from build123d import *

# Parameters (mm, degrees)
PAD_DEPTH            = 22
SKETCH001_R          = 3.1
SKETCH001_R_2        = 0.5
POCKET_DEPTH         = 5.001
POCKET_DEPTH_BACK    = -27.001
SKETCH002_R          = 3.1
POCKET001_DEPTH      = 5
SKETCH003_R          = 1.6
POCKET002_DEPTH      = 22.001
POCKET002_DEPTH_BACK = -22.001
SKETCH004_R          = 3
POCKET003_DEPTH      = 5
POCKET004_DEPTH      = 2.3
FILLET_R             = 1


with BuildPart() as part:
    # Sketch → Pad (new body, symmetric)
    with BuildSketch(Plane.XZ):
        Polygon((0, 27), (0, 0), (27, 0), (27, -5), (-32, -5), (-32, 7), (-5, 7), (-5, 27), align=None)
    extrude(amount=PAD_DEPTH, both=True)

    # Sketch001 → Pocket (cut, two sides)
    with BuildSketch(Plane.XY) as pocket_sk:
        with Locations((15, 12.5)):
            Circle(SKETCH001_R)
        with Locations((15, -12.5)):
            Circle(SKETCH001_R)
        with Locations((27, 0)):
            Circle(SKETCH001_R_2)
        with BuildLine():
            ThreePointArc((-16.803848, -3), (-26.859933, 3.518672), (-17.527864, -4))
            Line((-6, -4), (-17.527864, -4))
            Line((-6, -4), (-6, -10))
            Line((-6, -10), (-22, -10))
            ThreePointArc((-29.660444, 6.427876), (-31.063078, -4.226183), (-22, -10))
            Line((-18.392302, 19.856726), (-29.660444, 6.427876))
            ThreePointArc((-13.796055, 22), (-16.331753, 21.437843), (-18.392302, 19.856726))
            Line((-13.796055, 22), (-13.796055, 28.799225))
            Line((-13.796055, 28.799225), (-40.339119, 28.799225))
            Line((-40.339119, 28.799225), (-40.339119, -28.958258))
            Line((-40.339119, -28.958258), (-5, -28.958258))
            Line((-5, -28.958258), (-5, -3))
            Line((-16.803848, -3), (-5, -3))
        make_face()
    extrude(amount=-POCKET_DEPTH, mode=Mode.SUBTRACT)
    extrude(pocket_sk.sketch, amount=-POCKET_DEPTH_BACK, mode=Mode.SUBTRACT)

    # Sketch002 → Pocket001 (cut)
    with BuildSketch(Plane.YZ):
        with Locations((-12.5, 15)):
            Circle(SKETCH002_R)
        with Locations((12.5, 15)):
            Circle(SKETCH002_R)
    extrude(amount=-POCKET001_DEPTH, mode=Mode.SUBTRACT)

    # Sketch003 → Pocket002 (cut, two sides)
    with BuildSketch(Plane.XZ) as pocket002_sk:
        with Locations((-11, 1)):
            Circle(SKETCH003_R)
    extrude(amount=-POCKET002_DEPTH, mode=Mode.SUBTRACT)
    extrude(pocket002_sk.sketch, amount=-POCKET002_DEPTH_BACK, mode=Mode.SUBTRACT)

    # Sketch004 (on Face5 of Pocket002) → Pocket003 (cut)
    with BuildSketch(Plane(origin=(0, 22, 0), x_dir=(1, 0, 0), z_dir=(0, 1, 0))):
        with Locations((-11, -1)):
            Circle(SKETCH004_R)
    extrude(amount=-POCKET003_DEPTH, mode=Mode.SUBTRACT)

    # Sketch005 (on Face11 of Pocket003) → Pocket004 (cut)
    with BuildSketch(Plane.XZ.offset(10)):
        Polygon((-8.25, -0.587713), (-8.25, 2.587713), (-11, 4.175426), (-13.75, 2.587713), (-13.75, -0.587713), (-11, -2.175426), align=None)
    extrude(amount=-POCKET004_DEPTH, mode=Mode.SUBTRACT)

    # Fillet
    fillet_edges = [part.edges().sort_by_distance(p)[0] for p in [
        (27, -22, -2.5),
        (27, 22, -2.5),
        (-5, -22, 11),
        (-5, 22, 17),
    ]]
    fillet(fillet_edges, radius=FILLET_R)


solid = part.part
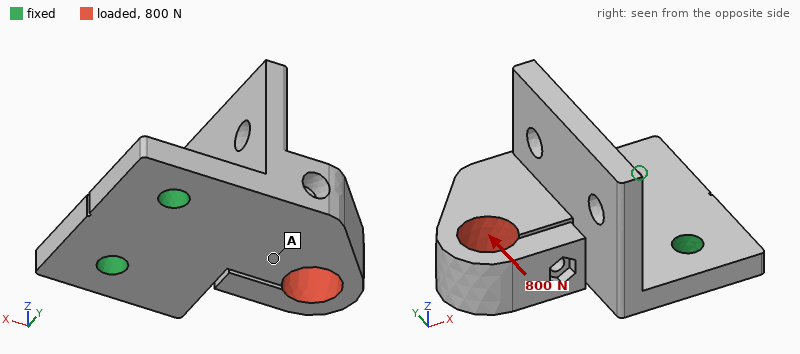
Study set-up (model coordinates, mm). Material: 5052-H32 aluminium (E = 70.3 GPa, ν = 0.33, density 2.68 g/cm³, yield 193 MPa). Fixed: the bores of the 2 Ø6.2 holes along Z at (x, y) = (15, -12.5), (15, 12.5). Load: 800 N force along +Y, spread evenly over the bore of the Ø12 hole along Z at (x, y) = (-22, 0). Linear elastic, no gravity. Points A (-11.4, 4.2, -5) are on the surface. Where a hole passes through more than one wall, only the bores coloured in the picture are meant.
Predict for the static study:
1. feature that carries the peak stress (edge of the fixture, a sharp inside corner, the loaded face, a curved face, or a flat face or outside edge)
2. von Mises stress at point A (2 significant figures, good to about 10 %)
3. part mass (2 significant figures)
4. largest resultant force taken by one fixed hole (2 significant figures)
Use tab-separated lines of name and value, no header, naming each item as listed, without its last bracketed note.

feature that carries the peak stress	the loaded face
von Mises stress at point A	14 MPa
part mass	50 g
largest resultant force taken by one fixed hole	1.2 kN
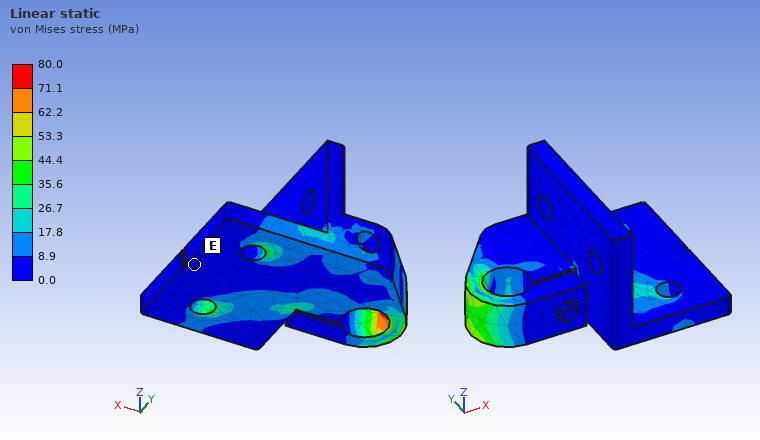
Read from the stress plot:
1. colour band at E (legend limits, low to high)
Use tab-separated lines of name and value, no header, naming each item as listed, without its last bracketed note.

colour band at E	0.0 to 8.9 MPa
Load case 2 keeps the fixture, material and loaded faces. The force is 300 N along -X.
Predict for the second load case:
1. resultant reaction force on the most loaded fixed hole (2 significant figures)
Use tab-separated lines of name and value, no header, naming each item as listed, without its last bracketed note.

resultant reaction force on the most loaded fixed hole	160 N
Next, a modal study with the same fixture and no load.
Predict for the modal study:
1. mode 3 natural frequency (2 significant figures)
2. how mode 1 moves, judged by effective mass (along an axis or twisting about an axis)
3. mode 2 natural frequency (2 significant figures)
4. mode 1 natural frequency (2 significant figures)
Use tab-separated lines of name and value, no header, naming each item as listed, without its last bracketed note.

mode 3 natural frequency	3300 Hz
how mode 1 moves, judged by effective mass	along Z
mode 2 natural frequency	2500 Hz
mode 1 natural frequency	1700 Hz
